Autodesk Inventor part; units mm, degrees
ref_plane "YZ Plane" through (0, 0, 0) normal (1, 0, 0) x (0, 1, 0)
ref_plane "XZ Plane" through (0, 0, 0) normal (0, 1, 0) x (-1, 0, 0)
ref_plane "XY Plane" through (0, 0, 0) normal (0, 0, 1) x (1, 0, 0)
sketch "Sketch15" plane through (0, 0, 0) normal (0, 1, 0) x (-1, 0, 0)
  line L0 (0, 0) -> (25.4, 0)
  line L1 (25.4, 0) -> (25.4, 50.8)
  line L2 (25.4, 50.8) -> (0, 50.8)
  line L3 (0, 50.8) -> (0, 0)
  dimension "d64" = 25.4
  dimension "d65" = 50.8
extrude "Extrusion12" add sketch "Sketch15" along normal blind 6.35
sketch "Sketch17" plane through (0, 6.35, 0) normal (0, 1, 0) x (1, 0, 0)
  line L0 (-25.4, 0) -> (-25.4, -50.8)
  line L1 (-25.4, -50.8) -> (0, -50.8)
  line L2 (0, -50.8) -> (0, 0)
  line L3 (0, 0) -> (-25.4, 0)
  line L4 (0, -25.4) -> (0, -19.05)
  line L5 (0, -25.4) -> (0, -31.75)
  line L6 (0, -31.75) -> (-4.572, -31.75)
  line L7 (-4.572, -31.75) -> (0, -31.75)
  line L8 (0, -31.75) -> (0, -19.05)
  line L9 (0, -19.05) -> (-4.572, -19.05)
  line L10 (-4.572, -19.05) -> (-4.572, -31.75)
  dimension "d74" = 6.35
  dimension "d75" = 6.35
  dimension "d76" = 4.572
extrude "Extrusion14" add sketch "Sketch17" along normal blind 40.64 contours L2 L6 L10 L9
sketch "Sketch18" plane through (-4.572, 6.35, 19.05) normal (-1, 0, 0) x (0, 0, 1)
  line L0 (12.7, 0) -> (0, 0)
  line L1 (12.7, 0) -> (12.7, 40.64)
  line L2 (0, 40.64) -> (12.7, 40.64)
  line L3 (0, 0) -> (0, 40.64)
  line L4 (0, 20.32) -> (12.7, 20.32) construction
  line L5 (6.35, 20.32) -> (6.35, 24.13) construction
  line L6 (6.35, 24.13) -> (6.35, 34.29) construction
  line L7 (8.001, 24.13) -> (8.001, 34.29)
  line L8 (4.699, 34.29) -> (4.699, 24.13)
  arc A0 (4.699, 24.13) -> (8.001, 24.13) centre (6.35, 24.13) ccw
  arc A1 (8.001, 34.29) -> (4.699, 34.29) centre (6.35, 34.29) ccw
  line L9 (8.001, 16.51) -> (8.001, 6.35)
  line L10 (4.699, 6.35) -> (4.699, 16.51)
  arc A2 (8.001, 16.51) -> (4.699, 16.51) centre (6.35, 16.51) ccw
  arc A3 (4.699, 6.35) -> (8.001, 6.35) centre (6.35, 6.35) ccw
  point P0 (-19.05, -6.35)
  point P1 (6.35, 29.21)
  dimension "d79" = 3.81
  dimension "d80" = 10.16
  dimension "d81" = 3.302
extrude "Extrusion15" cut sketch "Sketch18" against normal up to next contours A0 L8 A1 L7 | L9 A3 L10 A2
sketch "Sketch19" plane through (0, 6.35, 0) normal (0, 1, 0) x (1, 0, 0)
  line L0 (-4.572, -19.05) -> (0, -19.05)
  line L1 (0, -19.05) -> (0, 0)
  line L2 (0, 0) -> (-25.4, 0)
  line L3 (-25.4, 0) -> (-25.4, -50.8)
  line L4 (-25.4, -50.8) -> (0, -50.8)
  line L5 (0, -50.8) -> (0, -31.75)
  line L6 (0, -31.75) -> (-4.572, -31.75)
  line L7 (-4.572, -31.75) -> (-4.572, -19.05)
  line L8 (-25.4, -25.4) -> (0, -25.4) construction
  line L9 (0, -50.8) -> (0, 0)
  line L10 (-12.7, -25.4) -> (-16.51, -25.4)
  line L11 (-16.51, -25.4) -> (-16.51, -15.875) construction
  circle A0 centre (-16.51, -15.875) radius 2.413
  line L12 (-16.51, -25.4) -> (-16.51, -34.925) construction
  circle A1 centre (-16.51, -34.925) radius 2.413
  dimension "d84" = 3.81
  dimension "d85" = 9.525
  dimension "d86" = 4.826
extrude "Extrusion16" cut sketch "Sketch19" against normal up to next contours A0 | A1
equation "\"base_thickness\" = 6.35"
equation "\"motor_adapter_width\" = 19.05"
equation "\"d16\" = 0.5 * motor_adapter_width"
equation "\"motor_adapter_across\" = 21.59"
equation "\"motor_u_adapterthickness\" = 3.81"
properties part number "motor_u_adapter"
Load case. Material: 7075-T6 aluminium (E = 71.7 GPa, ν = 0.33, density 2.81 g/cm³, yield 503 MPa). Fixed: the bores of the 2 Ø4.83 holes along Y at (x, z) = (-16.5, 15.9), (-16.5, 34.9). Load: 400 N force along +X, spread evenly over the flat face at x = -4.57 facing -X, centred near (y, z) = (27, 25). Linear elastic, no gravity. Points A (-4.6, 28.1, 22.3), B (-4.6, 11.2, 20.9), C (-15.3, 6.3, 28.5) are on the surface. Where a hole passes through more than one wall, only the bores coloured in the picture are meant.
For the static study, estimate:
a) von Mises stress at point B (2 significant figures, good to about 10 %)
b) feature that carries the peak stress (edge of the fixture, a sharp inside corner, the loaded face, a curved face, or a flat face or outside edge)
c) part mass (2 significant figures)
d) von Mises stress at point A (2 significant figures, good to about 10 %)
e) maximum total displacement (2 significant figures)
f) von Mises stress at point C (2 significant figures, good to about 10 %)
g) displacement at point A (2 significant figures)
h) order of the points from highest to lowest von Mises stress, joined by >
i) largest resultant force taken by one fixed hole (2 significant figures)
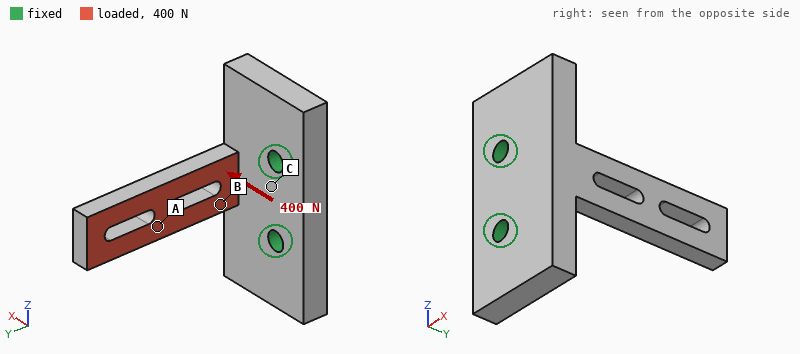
170 MPa
the loaded face
28 g
50 MPa
0.77 mm
21 MPa
0.33 mm
B > A > C
220 N
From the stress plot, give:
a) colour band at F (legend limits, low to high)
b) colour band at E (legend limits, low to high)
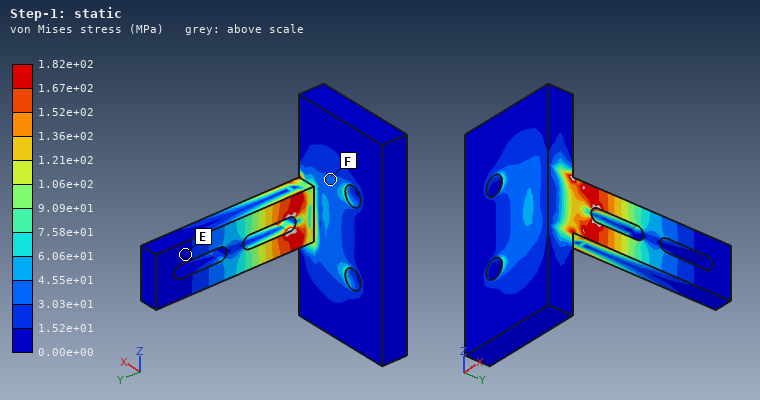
3.03e+01 to 4.55e+01 MPa
0.00e+00 to 1.52e+01 MPa
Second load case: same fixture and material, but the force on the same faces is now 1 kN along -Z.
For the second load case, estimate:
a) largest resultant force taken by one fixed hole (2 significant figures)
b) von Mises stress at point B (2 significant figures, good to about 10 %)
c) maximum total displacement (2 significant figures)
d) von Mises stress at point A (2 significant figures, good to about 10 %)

1.3 kN
130 MPa
0.44 mm
44 MPa
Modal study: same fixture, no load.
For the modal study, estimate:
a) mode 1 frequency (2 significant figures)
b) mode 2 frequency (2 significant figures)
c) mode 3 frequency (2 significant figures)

1900 Hz
4000 Hz
9100 Hz
